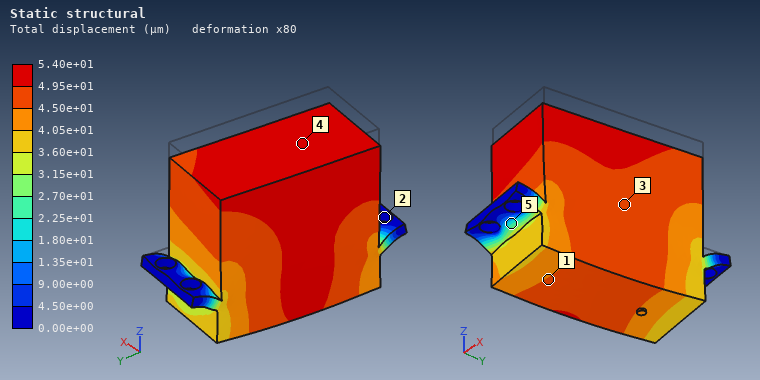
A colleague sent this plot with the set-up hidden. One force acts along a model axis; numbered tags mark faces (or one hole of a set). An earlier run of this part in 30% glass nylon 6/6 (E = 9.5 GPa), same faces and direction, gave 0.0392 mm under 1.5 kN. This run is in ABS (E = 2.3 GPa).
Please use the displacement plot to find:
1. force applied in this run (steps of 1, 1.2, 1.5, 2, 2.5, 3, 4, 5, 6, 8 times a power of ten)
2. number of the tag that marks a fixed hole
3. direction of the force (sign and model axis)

500 N
2
-Z
